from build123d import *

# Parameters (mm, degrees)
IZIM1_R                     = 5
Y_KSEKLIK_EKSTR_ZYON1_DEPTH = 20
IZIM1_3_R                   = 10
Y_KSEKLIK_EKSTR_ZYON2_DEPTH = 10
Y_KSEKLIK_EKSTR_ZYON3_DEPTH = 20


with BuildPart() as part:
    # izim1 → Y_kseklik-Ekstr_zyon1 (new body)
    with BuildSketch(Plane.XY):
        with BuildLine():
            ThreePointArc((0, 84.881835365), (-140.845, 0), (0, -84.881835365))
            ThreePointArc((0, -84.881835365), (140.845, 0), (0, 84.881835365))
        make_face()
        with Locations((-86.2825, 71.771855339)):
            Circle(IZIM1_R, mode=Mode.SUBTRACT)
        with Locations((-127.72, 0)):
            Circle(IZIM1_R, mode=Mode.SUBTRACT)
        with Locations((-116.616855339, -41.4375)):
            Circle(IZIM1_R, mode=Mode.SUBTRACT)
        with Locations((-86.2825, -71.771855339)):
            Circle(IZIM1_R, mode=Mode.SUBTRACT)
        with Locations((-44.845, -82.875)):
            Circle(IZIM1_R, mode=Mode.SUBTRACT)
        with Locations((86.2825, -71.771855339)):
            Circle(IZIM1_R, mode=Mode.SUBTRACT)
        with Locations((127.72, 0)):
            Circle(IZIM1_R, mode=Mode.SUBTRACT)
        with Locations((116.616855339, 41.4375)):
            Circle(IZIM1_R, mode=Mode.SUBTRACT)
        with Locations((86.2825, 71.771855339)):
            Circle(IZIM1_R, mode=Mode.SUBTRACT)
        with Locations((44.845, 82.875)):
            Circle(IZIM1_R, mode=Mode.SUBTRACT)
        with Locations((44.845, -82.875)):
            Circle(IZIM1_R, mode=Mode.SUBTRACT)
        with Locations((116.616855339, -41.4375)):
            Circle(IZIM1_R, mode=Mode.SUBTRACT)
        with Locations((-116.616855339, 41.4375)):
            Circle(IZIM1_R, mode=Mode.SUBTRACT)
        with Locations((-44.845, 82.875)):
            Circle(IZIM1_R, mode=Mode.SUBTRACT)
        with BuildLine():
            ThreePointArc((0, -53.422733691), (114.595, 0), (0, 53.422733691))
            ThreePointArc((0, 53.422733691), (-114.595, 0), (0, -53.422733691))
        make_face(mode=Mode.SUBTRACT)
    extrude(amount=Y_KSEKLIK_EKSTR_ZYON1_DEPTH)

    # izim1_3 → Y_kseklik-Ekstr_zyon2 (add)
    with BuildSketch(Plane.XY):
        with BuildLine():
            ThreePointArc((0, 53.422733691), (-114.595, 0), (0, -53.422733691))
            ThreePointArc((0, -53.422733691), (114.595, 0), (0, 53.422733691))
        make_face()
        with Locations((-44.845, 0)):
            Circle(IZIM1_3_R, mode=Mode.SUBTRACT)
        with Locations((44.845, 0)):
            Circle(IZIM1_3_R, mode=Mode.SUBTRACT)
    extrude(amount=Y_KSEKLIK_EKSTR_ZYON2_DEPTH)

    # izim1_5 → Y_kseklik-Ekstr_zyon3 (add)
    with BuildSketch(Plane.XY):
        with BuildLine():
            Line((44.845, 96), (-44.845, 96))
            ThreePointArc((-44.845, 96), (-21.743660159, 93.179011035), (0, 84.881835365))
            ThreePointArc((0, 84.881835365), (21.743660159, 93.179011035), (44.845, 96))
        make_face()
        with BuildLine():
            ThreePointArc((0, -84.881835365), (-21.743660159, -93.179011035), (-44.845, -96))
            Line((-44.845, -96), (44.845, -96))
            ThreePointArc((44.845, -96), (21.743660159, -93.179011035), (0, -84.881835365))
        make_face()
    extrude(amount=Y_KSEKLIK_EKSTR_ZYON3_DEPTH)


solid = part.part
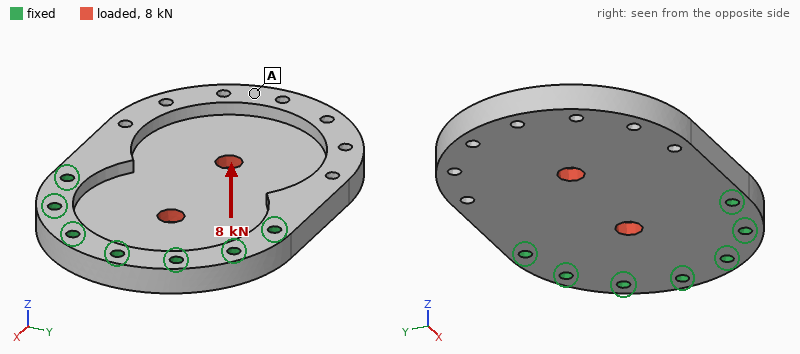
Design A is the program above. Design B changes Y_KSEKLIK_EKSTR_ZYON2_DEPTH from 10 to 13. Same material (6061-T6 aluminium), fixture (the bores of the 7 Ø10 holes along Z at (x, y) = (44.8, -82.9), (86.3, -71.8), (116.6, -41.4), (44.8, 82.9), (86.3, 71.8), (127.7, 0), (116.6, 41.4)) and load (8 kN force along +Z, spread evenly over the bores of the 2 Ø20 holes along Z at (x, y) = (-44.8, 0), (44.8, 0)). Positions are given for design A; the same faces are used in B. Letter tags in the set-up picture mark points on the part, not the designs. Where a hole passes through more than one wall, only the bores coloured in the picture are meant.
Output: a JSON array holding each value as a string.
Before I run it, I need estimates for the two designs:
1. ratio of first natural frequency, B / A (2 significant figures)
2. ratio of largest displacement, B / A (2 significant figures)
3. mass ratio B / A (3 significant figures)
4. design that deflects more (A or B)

["1.0", "0.92", "1.13", "A"]
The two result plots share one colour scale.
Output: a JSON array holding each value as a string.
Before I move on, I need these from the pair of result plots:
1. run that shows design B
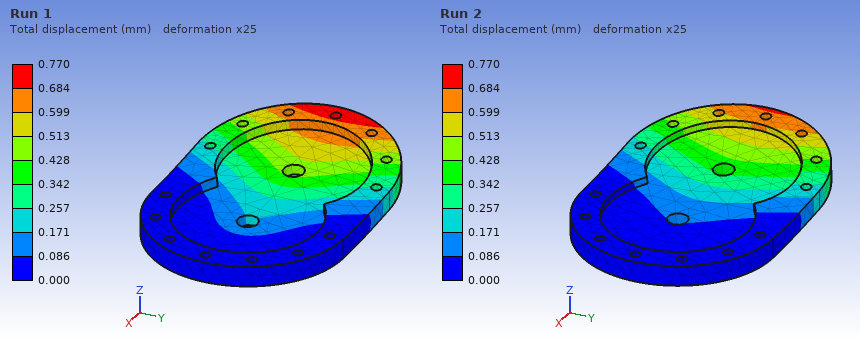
["Run 2"]
